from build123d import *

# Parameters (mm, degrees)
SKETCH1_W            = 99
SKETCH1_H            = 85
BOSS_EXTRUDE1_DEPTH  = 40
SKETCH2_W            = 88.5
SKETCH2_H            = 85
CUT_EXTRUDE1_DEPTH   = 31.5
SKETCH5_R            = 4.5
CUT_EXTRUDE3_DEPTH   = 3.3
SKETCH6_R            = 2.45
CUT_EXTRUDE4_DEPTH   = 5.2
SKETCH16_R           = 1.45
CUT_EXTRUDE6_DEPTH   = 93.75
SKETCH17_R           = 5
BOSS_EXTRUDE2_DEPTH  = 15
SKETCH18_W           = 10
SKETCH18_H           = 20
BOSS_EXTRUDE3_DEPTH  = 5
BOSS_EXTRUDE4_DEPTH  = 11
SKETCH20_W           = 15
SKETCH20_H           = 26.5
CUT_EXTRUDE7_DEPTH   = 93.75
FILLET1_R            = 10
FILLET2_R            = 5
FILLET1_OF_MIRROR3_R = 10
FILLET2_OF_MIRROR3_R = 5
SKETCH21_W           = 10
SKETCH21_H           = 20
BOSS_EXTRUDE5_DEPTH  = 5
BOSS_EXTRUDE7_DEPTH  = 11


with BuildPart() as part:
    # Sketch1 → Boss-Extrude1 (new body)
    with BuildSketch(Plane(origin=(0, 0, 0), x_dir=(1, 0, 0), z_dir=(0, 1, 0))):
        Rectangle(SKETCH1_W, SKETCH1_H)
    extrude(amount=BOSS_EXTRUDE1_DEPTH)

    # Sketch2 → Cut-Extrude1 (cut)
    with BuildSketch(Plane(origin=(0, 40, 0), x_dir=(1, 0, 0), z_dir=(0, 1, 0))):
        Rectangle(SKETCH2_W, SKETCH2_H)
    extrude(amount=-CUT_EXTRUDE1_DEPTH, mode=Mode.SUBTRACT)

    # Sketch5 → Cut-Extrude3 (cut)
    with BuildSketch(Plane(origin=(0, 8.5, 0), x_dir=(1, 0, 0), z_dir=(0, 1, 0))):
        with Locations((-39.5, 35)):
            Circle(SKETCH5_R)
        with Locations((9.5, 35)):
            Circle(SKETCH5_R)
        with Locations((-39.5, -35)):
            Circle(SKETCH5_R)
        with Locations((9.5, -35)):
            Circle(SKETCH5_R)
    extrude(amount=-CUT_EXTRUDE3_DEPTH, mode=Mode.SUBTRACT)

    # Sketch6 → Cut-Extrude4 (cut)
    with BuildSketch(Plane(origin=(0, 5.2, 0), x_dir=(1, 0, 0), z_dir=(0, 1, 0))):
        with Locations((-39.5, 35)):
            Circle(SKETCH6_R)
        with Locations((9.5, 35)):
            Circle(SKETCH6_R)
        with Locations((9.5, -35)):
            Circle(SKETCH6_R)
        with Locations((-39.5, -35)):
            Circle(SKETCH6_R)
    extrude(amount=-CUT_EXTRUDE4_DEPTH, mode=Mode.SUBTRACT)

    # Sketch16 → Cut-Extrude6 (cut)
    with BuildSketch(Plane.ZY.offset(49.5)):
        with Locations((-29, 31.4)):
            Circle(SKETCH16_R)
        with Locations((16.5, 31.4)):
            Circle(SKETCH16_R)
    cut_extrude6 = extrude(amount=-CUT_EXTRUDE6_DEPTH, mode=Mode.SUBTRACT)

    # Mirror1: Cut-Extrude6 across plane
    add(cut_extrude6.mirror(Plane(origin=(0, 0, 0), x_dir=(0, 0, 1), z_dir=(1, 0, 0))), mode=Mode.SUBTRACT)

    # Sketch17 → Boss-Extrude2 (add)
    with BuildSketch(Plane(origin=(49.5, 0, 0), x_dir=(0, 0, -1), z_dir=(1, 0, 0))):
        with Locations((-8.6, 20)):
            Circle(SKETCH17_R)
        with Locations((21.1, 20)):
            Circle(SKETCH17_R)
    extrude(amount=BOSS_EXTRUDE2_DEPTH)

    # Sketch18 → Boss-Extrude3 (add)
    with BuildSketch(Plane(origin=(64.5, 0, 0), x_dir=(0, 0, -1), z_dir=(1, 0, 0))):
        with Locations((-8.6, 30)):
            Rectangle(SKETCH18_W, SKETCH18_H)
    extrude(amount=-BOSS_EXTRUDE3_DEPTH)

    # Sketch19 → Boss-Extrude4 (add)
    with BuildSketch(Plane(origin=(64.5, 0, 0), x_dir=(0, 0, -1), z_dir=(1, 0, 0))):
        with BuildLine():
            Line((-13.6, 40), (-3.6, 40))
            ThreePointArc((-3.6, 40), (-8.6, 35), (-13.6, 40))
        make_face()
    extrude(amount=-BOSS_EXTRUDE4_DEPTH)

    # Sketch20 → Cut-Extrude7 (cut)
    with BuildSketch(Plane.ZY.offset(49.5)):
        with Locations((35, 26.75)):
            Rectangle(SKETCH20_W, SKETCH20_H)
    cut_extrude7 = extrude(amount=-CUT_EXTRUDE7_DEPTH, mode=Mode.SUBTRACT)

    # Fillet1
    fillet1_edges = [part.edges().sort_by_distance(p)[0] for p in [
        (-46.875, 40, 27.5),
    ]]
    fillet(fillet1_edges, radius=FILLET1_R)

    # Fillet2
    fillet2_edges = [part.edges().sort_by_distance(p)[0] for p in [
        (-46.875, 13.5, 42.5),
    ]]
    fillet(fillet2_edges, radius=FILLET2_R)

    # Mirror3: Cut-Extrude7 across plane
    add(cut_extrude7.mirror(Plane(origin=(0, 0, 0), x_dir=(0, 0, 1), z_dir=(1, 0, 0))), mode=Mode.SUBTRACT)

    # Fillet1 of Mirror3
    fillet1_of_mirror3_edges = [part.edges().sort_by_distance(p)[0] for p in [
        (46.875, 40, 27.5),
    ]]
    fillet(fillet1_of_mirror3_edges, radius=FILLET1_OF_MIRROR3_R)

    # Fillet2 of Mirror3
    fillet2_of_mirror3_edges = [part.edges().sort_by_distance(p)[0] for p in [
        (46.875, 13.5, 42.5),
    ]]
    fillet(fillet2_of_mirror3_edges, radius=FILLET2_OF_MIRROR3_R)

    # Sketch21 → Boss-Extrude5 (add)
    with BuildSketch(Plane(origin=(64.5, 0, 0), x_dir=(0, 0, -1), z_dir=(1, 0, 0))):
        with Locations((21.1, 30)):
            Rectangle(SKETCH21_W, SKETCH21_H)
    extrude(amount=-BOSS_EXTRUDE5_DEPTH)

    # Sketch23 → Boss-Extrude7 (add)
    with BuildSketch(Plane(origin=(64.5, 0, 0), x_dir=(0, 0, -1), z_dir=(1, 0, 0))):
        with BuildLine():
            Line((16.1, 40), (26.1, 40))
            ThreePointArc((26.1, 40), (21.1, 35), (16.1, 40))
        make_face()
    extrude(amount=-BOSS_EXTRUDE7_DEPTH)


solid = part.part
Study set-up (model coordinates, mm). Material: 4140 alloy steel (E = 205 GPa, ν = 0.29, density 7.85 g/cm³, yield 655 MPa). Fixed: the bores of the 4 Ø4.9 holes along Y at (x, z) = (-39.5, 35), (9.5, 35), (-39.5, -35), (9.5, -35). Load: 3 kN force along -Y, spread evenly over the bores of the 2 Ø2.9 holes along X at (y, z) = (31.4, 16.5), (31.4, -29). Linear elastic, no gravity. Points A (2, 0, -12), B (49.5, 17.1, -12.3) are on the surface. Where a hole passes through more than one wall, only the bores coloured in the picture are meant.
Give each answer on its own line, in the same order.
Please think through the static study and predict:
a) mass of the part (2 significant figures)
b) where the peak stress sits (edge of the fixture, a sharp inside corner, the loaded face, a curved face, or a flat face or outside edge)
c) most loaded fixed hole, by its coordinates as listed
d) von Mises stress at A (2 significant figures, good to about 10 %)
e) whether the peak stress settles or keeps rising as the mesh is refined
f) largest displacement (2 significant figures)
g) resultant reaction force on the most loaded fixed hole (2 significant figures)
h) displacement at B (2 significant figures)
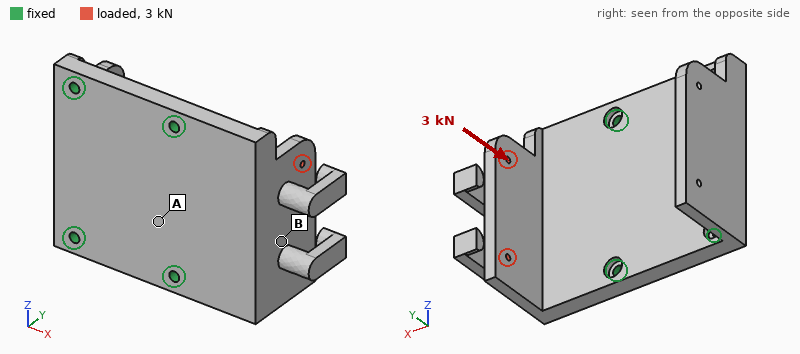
770 g
edge of the fixture
(9.5, -35)
53 MPa
keeps rising
0.23 mm
3.1 kN
0.13 mm
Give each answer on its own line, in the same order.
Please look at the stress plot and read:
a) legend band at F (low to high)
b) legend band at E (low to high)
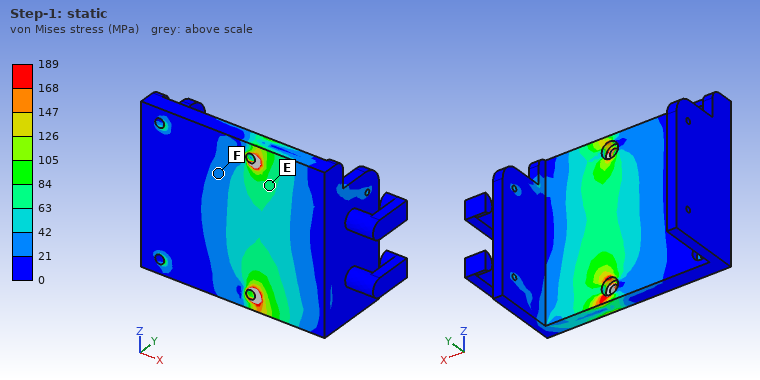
21 to 42 MPa
63 to 84 MPa
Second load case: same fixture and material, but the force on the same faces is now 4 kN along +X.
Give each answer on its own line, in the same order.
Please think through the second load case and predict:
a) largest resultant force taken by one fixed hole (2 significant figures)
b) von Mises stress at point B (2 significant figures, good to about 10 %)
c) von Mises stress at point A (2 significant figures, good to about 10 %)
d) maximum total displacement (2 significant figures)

2.1 kN
140 MPa
51 MPa
0.48 mm
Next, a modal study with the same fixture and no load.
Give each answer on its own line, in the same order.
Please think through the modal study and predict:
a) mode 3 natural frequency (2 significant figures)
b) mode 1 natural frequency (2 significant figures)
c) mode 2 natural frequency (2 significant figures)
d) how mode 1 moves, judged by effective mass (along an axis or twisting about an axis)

3200 Hz
1400 Hz
3000 Hz
along Y
